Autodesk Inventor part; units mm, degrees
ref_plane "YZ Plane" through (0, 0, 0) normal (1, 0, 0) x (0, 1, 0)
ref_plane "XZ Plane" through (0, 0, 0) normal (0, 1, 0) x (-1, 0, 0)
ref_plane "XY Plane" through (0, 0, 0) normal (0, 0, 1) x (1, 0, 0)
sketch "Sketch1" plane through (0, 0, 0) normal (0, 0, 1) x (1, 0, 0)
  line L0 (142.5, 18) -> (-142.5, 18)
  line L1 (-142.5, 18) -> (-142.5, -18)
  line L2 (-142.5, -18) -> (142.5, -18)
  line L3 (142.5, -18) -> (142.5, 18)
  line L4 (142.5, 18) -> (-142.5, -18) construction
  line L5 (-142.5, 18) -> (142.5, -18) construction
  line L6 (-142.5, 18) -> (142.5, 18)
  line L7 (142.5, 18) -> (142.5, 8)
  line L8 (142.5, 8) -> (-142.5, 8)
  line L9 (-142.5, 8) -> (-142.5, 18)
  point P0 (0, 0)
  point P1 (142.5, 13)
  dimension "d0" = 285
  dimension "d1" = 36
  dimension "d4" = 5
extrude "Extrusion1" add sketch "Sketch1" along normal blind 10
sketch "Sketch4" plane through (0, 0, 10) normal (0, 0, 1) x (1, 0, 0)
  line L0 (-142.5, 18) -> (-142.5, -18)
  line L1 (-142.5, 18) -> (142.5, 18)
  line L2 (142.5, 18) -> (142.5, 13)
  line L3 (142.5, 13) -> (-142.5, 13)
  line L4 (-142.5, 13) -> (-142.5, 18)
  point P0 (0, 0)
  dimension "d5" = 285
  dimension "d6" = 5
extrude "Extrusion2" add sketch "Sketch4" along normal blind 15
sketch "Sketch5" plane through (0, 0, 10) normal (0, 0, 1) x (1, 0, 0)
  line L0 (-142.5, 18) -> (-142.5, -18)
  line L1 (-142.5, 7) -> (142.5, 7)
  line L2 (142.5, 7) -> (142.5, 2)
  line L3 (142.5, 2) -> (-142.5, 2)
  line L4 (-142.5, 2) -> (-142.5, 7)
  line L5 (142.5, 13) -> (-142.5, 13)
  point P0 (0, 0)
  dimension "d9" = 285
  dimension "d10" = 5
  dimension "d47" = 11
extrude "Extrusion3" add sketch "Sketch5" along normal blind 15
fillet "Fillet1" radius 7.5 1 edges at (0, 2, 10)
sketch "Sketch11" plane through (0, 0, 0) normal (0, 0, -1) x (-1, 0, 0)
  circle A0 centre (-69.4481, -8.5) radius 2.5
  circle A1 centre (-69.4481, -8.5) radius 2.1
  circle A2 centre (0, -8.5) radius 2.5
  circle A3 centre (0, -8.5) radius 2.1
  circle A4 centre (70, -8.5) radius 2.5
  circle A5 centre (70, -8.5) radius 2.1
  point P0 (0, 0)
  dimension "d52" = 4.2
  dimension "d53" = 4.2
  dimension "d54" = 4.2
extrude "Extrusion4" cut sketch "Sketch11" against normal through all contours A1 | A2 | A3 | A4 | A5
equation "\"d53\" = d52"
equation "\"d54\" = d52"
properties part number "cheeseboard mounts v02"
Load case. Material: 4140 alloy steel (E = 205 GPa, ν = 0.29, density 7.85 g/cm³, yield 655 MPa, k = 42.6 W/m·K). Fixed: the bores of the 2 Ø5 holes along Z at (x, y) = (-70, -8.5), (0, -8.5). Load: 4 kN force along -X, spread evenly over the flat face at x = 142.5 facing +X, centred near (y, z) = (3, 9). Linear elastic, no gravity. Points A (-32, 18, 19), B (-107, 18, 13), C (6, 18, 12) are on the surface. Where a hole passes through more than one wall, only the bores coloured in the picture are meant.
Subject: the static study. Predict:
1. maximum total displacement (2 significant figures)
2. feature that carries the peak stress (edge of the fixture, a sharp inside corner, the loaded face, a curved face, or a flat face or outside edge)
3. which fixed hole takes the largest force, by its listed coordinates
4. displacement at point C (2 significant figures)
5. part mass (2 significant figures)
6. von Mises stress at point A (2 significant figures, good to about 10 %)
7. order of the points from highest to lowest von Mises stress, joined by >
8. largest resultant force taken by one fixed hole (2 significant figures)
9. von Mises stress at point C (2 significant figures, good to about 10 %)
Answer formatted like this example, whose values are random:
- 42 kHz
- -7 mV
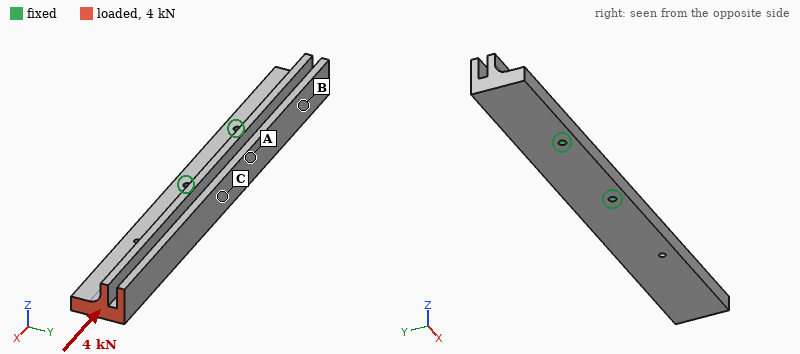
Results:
- 14 µm
- edge of the fixture
- (0, -8.5)
- 2.9 µm
- 1.2 kg
- 5.1 MPa
- C > A > B
- 2.9 kN
- 8.6 MPa
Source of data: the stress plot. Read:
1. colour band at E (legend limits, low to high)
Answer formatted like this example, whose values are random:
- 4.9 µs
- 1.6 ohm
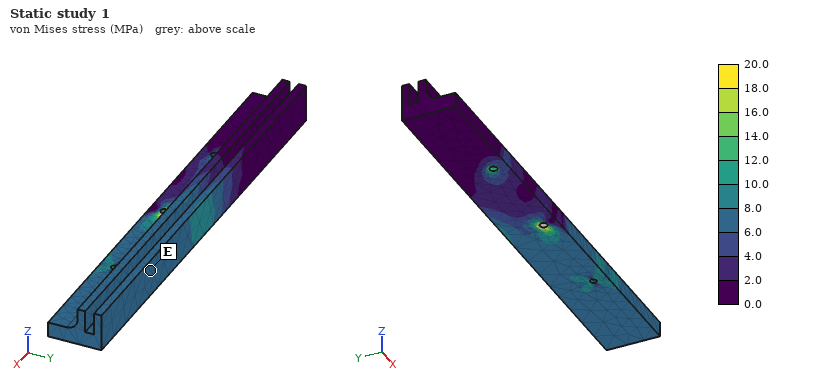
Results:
- 6.0 to 8.0 MPa
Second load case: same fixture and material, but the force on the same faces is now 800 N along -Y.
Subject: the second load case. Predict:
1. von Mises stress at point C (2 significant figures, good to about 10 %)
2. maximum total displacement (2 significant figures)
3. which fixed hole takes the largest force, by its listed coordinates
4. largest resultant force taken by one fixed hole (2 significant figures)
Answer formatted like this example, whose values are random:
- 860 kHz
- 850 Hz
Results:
- 28 MPa
- 0.15 mm
- (0, -8.5)
- 3.0 kN
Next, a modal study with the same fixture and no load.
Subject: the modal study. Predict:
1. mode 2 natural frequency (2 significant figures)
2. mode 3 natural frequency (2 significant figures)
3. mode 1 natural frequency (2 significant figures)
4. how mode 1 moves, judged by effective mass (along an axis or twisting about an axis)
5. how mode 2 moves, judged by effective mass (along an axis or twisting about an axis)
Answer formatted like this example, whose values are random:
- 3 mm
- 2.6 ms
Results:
- 1100 Hz
- 2000 Hz
- 640 Hz
- along Z
- along Y
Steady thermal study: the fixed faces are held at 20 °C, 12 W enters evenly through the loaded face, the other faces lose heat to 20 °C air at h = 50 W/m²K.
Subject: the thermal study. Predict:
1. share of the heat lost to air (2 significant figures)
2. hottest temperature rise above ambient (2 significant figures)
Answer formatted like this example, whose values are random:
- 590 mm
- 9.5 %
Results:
- 89 %
- 30 K
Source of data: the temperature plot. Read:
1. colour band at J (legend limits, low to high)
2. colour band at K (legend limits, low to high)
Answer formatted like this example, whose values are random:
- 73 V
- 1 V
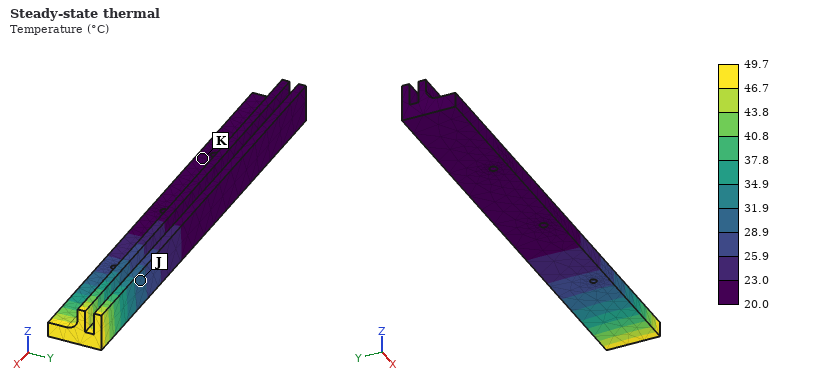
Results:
- 28.9 to 31.9 °C
- 20.0 to 23.0 °C
